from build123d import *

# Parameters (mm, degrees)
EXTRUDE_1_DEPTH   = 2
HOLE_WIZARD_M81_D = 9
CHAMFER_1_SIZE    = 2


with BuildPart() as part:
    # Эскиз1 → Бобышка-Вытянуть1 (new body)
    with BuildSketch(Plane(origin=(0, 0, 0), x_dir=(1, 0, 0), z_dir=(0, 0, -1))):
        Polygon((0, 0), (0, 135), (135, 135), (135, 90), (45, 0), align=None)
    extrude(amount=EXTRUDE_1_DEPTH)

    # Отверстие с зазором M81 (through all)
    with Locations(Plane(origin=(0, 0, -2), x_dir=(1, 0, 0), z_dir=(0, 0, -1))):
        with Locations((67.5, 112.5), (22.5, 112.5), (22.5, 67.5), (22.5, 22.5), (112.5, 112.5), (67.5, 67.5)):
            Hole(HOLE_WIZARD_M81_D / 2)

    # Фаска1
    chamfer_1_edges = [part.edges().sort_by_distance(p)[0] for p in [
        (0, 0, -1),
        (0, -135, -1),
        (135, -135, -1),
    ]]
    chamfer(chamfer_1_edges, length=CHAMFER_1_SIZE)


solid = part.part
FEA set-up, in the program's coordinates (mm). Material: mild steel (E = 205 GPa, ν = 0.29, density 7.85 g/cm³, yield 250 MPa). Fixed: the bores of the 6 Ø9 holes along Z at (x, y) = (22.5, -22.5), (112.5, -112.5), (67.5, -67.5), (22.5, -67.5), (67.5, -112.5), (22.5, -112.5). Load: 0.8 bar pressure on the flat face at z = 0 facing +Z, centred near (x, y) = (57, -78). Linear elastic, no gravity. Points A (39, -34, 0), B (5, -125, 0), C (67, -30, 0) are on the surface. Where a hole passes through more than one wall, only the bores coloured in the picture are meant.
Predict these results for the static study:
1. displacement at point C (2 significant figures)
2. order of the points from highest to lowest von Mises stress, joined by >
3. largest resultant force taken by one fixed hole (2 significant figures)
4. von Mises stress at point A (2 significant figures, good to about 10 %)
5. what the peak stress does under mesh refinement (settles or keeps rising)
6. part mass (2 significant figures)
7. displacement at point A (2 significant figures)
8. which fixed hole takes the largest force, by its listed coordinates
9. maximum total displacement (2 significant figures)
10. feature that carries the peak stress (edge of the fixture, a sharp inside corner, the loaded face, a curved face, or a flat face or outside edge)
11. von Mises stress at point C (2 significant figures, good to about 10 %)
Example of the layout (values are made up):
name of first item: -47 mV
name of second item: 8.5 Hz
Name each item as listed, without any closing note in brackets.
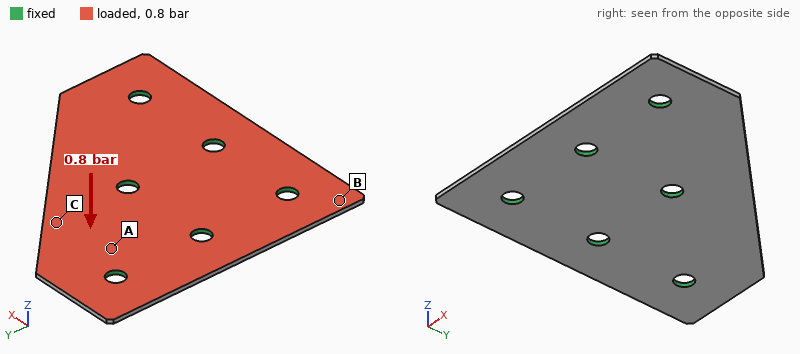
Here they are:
displacement at point C: 70 µm
order of the points from highest to lowest von Mises stress, joined by >: A > C > B
largest resultant force taken by one fixed hole: 260 N
von Mises stress at point A: 22 MPa
what the peak stress does under mesh refinement: keeps rising
part mass: 220 g
displacement at point A: 16 µm
which fixed hole takes the largest force, by its listed coordinates: (67.5, -67.5)
maximum total displacement: 85 µm
feature that carries the peak stress: edge of the fixture
von Mises stress at point C: 15 MPa
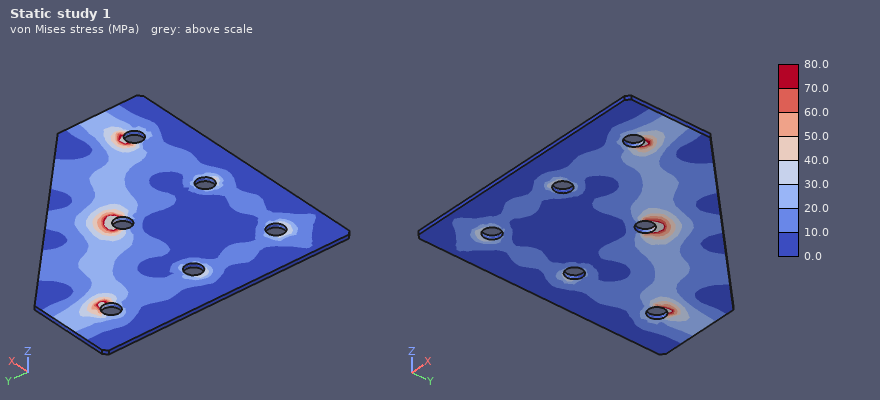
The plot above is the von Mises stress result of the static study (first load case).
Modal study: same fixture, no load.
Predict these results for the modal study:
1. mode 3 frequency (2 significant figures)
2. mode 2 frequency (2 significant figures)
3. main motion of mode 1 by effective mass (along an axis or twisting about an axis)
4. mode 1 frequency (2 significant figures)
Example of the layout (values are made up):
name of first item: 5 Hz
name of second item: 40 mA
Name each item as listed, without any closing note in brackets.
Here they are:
mode 3 frequency: 3000 Hz
mode 2 frequency: 1800 Hz
main motion of mode 1 by effective mass: along Z
mode 1 frequency: 1600 Hz
